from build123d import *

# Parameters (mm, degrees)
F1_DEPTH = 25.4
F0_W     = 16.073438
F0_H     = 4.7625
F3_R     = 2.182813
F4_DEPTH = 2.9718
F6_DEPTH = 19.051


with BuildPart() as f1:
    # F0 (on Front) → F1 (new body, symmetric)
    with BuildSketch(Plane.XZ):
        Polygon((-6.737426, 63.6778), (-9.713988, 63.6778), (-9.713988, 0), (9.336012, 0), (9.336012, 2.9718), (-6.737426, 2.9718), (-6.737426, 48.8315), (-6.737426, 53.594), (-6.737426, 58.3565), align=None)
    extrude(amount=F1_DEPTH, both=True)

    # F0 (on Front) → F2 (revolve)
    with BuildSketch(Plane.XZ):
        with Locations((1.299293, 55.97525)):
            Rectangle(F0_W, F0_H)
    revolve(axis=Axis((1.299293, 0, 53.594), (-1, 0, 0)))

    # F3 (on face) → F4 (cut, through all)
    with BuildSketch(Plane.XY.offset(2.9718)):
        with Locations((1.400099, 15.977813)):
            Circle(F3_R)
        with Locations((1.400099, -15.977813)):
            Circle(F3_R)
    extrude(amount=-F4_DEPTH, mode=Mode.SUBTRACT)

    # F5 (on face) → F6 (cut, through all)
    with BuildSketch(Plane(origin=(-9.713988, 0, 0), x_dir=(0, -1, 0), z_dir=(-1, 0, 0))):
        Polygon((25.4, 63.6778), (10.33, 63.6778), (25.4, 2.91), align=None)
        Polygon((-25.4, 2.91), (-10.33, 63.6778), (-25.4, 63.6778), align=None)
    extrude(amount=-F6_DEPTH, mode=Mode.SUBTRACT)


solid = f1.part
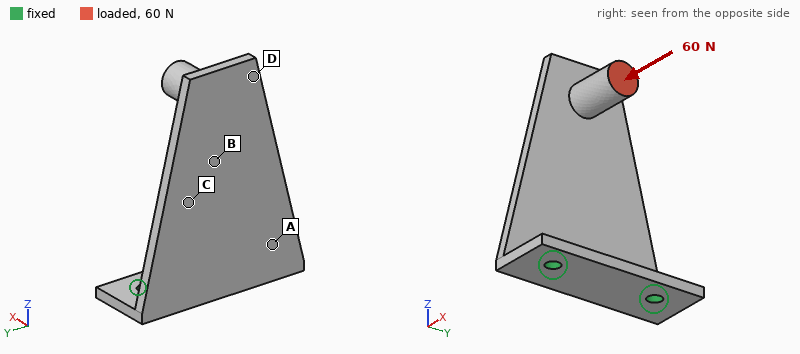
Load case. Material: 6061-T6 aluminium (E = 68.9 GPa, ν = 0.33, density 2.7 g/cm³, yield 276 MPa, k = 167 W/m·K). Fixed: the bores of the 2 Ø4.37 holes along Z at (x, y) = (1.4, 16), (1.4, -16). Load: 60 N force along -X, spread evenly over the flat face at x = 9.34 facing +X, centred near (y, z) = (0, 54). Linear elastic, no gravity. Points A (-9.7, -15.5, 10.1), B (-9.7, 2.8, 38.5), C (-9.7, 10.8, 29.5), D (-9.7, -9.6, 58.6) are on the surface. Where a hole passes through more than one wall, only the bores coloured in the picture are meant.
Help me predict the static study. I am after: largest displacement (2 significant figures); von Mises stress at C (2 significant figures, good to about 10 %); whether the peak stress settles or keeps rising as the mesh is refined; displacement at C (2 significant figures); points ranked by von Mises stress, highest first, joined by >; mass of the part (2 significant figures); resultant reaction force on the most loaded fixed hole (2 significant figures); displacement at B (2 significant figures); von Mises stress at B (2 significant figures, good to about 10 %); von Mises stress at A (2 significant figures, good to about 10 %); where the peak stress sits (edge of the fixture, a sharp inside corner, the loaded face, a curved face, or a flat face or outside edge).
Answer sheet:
0.76 mm
26 MPa
keeps rising
0.24 mm
A > C > B > D
28 g
34 N
0.36 mm
19 MPa
35 MPa
edge of the fixture
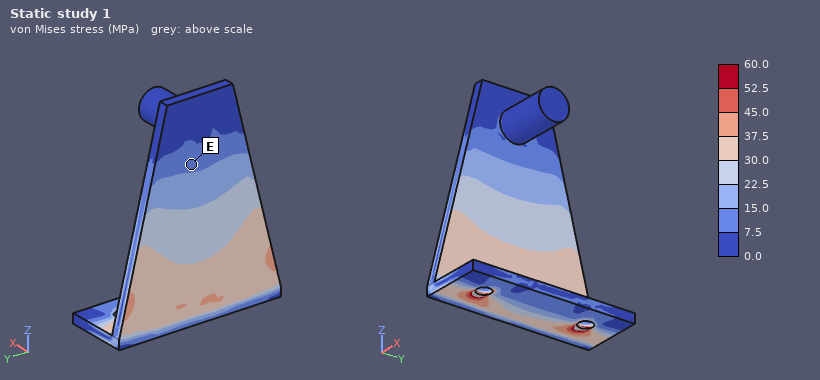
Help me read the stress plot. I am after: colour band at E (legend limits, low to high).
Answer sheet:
7.5 to 15.0 MPa
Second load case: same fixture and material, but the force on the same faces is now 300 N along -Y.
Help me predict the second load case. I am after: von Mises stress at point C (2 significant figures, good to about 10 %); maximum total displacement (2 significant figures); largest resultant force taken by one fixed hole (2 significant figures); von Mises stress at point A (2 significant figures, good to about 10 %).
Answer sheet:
78 MPa
0.73 mm
480 N
57 MPa
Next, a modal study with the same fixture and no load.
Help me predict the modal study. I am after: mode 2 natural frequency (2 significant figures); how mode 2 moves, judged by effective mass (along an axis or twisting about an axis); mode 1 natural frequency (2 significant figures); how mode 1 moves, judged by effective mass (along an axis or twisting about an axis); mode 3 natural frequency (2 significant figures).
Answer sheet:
2000 Hz
along Y
530 Hz
along X
2800 Hz
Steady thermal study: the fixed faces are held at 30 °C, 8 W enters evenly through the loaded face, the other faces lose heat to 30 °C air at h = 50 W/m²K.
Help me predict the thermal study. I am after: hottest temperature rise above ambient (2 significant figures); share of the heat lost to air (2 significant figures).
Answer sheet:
30 K
38 %
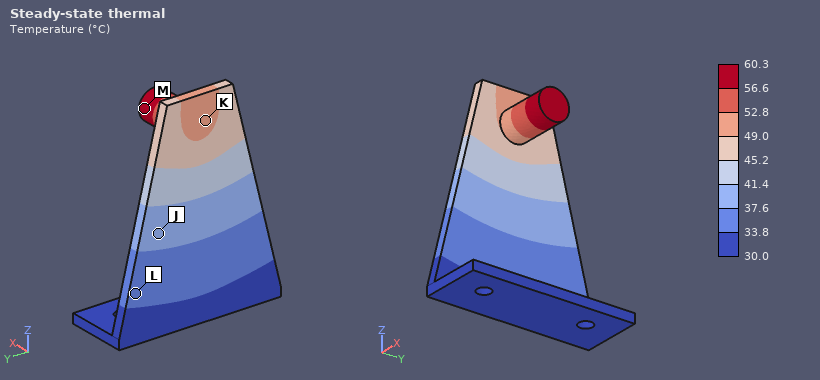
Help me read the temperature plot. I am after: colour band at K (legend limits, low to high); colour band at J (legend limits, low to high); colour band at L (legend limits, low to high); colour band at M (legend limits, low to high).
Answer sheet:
49.0 to 52.8 °C
37.6 to 41.4 °C
33.8 to 37.6 °C
56.6 to 60.3 °C
